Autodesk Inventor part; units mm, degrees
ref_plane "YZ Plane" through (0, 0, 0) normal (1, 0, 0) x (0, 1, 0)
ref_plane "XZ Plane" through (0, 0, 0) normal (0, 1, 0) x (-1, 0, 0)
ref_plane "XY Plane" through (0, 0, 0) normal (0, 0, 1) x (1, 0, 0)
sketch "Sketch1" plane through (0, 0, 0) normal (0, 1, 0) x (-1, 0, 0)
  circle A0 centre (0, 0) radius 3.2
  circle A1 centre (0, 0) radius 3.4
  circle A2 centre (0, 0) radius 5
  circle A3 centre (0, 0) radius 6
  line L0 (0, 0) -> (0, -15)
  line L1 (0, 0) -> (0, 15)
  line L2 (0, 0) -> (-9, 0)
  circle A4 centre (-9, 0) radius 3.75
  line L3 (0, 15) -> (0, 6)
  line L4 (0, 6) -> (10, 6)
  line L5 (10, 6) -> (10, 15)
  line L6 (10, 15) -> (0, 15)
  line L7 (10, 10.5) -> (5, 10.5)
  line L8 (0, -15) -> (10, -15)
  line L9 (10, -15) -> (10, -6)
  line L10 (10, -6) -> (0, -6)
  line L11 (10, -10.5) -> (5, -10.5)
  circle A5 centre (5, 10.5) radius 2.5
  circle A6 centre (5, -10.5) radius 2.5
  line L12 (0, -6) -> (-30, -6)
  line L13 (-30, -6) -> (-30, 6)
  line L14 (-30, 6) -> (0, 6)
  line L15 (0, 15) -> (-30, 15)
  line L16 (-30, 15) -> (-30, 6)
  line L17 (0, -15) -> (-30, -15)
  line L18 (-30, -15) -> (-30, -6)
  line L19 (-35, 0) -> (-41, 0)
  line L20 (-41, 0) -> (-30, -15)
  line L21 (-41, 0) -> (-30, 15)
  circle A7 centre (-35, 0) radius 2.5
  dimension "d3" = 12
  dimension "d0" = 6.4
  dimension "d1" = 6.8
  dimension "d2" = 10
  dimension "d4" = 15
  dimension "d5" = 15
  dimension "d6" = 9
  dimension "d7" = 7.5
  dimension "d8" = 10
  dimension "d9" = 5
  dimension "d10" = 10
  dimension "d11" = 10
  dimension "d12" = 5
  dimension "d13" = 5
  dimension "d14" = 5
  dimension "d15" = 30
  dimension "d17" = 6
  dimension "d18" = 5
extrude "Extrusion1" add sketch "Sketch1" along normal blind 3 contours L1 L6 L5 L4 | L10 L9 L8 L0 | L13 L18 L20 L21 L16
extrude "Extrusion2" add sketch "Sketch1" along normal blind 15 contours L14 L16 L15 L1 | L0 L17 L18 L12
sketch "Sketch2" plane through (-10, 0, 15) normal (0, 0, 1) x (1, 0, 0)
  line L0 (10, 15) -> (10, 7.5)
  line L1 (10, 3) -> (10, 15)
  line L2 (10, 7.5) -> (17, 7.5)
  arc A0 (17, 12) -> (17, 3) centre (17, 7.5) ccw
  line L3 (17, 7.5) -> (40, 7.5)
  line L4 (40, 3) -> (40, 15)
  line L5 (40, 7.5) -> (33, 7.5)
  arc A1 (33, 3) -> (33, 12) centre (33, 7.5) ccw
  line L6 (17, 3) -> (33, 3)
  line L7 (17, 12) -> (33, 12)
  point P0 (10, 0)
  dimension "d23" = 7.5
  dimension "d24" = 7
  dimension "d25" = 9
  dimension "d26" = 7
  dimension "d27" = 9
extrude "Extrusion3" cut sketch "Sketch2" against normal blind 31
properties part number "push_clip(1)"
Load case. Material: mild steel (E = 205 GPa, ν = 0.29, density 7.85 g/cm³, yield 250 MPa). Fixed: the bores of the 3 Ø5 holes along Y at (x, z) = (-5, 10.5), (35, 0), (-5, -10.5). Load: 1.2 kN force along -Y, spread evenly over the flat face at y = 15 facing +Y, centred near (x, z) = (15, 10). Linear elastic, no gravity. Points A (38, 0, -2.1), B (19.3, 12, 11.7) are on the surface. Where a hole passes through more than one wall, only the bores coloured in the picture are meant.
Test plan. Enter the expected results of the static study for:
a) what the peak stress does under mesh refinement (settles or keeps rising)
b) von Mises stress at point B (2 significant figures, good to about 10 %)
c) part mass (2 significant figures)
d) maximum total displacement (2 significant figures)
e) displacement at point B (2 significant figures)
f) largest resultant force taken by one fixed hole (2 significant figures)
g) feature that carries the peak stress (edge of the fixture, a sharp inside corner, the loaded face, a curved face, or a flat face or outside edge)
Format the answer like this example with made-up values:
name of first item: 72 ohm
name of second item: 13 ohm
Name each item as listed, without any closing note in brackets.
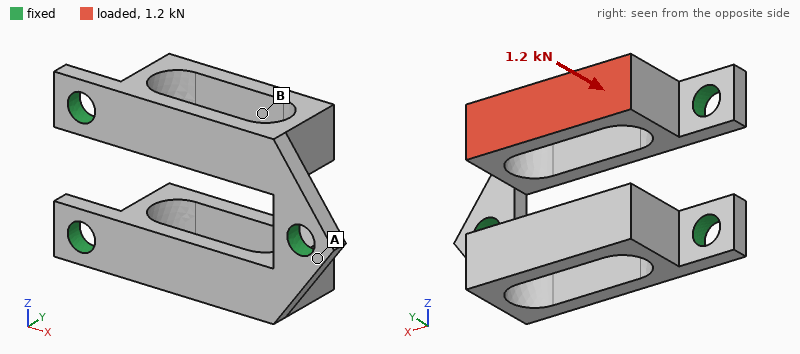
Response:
what the peak stress does under mesh refinement: keeps rising
von Mises stress at point B: 54 MPa
part mass: 41 g
maximum total displacement: 54 µm
displacement at point B: 41 µm
largest resultant force taken by one fixed hole: 660 N
feature that carries the peak stress: edge of the fixture
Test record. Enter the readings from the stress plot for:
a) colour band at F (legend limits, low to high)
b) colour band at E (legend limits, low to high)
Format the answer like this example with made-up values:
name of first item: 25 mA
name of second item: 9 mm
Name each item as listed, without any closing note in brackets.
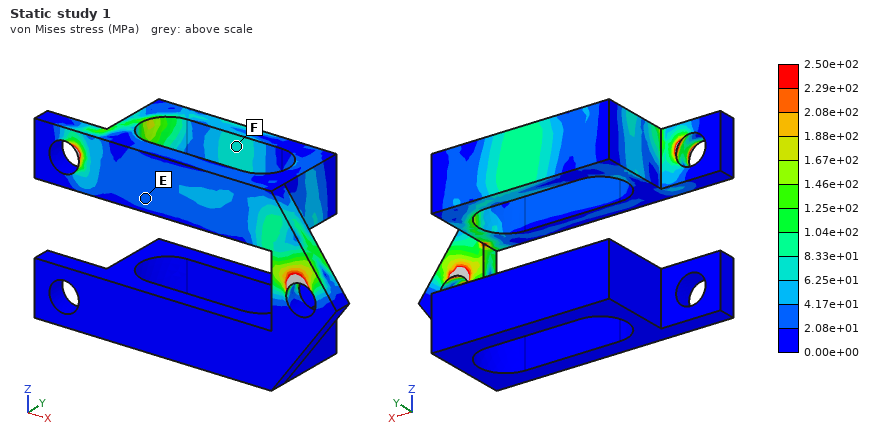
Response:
colour band at F: 6.25e+01 to 8.33e+01 MPa
colour band at E: 2.08e+01 to 4.17e+01 MPa
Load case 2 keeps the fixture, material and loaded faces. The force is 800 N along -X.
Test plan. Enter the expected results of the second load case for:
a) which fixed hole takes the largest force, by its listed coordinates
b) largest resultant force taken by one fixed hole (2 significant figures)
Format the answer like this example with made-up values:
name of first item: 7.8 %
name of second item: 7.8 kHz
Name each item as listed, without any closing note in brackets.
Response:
which fixed hole takes the largest force, by its listed coordinates: (-5, 10.5)
largest resultant force taken by one fixed hole: 680 N
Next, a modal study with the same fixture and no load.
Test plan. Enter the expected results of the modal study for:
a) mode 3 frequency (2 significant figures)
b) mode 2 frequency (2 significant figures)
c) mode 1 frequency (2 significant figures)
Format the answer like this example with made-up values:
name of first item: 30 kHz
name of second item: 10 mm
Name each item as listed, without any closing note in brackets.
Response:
mode 3 frequency: 10 kHz
mode 2 frequency: 5200 Hz
mode 1 frequency: 5200 Hz
